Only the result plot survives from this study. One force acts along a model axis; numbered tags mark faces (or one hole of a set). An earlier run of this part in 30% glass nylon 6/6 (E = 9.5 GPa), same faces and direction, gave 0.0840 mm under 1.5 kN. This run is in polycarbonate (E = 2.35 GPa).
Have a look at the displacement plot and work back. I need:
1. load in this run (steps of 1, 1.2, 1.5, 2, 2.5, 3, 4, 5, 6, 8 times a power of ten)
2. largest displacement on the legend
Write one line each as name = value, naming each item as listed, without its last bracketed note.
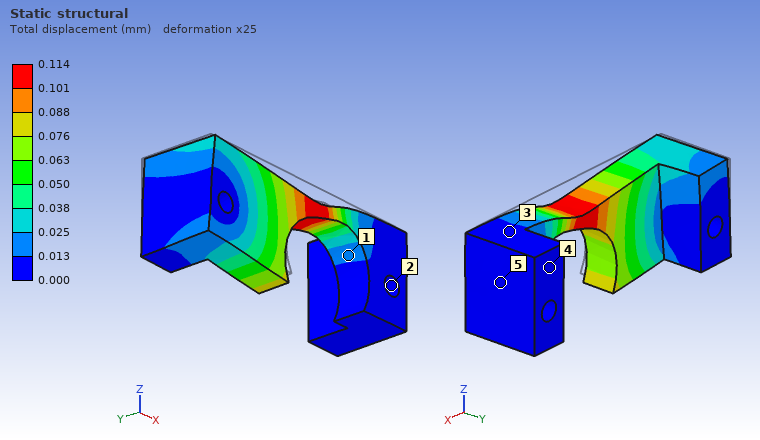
load in this run = 500 N
largest displacement on the legend = 0.114 mm
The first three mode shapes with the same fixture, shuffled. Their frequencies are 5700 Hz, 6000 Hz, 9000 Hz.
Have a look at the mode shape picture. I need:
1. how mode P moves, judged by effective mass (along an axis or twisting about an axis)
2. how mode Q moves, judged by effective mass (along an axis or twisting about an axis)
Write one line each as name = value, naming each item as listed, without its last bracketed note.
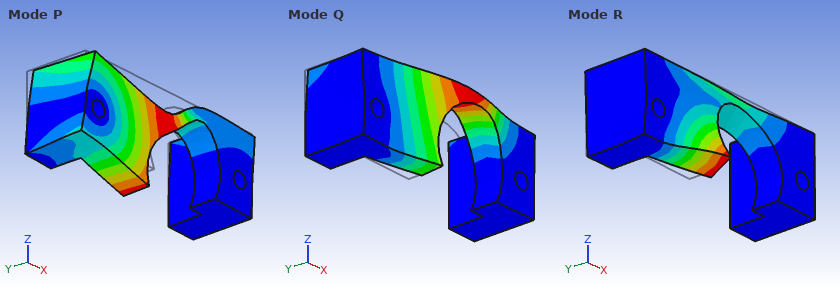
how mode P moves, judged by effective mass = along Z
how mode Q moves, judged by effective mass = along Y
